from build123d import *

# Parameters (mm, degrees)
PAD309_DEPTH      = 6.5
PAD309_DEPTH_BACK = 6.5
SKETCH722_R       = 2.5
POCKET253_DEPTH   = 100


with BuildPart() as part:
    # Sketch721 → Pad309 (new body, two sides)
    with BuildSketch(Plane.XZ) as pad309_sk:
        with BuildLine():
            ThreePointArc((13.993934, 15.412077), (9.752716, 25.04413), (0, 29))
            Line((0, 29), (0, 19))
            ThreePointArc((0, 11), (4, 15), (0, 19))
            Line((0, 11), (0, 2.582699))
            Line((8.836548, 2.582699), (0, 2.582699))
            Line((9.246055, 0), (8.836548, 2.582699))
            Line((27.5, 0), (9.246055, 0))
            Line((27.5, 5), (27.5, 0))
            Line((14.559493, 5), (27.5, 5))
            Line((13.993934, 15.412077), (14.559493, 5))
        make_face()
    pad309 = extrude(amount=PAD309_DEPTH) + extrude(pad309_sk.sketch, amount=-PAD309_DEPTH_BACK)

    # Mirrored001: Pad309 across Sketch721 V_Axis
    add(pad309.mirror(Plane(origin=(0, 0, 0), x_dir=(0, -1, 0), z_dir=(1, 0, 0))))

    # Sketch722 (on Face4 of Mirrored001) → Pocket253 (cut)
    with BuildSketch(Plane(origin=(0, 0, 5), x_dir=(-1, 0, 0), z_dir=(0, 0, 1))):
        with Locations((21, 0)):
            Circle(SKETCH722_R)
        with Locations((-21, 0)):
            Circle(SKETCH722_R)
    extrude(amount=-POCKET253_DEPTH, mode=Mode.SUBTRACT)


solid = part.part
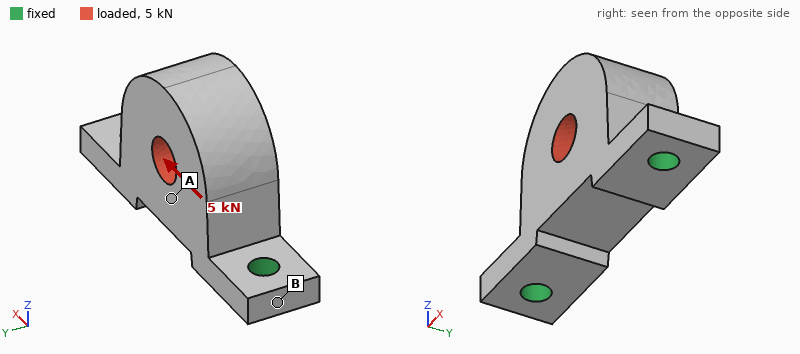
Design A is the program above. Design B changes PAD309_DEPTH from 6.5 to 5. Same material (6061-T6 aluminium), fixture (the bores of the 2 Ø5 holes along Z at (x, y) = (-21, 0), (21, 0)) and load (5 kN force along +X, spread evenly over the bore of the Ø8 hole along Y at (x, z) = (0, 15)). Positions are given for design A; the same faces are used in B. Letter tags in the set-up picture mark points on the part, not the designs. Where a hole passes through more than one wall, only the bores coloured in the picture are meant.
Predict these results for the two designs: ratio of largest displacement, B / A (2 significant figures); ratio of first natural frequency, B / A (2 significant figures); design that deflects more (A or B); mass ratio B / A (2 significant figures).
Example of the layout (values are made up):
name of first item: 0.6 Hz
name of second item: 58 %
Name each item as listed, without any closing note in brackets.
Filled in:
ratio of largest displacement, B / A: 1.1
ratio of first natural frequency, B / A: 0.97
design that deflects more: B
mass ratio B / A: 0.88
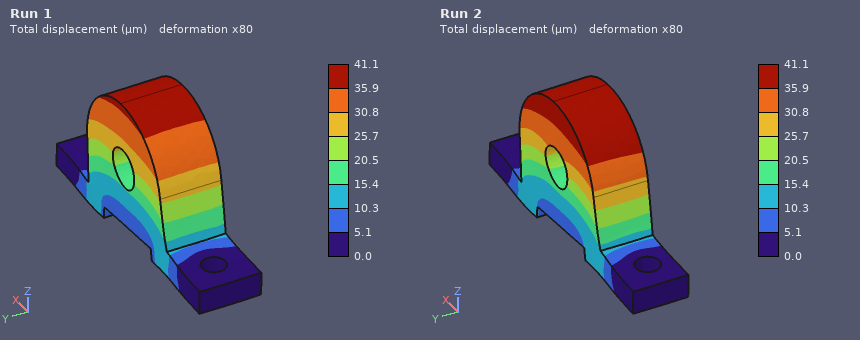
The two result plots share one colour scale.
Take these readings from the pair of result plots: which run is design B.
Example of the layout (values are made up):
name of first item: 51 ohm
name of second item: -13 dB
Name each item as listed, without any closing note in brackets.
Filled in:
which run is design B: Run 2
